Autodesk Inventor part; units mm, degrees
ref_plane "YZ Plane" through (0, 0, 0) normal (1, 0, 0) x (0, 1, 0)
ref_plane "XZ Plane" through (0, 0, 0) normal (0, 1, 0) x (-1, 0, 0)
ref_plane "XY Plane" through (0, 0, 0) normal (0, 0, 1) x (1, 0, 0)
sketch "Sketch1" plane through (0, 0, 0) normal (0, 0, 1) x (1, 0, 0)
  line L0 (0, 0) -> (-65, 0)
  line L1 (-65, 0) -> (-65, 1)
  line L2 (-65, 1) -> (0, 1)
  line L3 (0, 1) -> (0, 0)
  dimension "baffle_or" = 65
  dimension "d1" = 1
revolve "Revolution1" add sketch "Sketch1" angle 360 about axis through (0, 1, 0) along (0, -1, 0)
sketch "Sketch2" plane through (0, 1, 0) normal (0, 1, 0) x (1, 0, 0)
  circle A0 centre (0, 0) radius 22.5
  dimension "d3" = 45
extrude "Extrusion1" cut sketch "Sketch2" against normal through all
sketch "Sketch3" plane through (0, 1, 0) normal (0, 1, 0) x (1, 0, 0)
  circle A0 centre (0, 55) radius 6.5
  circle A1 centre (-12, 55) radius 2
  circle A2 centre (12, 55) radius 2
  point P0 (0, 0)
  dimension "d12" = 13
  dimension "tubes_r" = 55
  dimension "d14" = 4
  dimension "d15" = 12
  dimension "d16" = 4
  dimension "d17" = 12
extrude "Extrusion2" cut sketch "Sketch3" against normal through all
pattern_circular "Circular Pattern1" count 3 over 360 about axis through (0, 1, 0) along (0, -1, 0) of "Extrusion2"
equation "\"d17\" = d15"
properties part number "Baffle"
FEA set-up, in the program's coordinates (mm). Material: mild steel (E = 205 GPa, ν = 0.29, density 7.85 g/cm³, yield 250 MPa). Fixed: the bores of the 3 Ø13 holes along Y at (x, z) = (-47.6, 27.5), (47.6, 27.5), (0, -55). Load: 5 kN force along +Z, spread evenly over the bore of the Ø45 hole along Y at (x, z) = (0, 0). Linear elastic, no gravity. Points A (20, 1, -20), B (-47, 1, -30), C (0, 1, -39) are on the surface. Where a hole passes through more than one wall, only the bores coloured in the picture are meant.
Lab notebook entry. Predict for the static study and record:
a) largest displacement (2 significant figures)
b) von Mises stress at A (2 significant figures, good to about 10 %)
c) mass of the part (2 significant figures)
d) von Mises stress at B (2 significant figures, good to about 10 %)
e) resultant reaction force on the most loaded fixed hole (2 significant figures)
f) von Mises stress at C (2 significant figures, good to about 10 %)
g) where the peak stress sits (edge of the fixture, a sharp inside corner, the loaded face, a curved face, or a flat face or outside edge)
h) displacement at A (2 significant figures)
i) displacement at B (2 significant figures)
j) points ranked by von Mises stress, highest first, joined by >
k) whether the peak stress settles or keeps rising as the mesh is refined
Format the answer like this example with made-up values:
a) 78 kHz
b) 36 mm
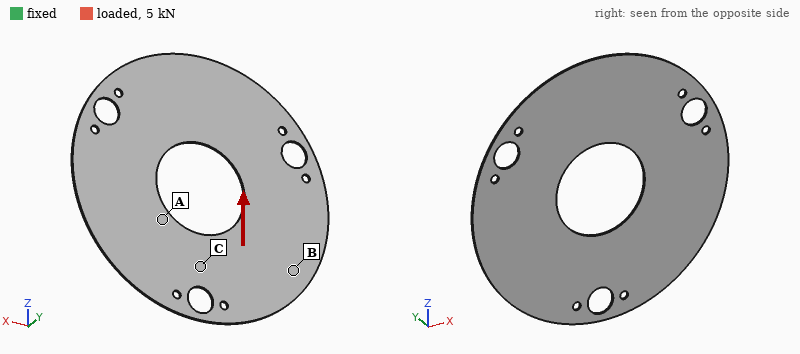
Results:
a) 17 µm
b) 43 MPa
c) 88 g
d) 16 MPa
e) 1.7 kN
f) 62 MPa
g) edge of the fixture
h) 9.2 µm
i) 7.2 µm
j) C > A > B
k) keeps rising
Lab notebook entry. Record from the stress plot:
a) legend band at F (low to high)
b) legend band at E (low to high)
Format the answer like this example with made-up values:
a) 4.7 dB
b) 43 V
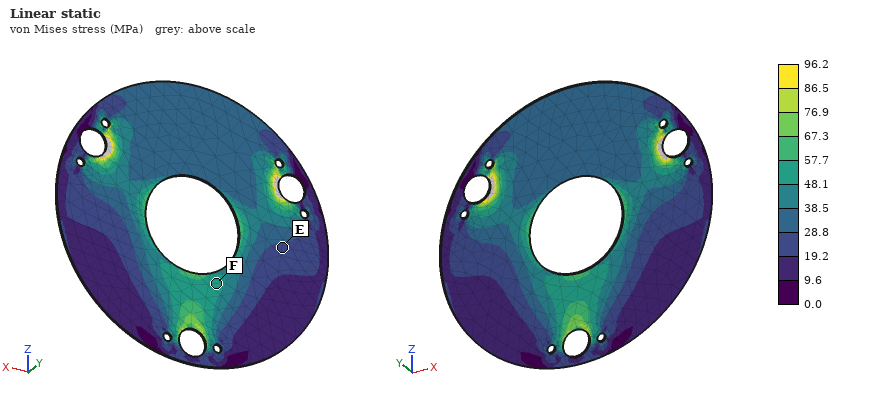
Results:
a) 48.1 to 57.7 MPa
b) 19.2 to 28.8 MPa
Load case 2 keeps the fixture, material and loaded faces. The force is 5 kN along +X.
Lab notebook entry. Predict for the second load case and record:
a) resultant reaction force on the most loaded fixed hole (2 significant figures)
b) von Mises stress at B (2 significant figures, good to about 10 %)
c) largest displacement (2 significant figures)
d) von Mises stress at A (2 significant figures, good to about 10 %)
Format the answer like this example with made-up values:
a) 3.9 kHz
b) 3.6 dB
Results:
a) 1.8 kN
b) 29 MPa
c) 16 µm
d) 32 MPa
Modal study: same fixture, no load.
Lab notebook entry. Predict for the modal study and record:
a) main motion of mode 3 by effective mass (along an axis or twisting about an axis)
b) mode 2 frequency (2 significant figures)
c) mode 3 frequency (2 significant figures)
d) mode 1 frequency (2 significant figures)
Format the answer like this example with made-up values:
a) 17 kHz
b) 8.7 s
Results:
a) along Y
b) 470 Hz
c) 500 Hz
d) 470 Hz
